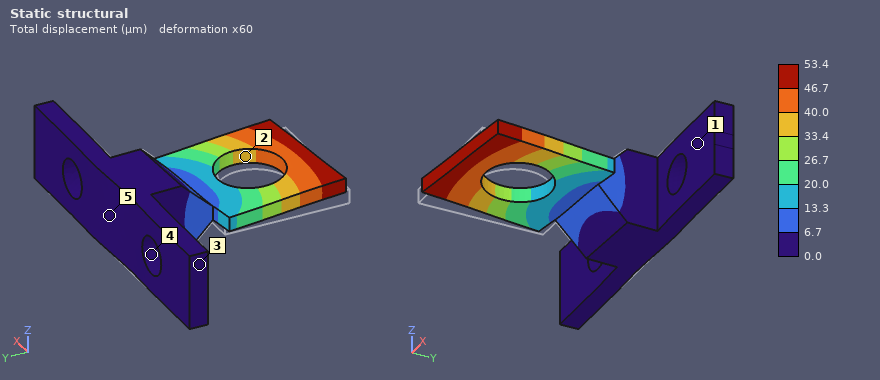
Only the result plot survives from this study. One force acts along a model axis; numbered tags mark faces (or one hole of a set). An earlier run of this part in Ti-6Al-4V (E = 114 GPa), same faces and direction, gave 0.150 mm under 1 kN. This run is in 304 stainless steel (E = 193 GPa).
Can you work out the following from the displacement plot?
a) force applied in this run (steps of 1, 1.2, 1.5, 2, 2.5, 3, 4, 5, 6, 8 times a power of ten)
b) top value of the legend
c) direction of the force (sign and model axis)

600 N
53.4 µm
+X
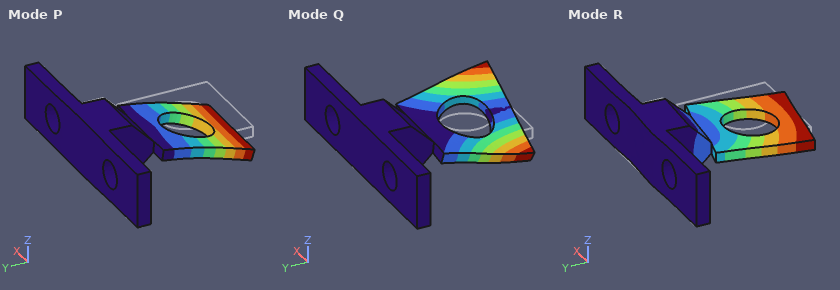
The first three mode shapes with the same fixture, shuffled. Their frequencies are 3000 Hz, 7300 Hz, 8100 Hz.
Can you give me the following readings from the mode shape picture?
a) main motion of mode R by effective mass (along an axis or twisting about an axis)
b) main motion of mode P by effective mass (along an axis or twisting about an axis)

along X
along Z
